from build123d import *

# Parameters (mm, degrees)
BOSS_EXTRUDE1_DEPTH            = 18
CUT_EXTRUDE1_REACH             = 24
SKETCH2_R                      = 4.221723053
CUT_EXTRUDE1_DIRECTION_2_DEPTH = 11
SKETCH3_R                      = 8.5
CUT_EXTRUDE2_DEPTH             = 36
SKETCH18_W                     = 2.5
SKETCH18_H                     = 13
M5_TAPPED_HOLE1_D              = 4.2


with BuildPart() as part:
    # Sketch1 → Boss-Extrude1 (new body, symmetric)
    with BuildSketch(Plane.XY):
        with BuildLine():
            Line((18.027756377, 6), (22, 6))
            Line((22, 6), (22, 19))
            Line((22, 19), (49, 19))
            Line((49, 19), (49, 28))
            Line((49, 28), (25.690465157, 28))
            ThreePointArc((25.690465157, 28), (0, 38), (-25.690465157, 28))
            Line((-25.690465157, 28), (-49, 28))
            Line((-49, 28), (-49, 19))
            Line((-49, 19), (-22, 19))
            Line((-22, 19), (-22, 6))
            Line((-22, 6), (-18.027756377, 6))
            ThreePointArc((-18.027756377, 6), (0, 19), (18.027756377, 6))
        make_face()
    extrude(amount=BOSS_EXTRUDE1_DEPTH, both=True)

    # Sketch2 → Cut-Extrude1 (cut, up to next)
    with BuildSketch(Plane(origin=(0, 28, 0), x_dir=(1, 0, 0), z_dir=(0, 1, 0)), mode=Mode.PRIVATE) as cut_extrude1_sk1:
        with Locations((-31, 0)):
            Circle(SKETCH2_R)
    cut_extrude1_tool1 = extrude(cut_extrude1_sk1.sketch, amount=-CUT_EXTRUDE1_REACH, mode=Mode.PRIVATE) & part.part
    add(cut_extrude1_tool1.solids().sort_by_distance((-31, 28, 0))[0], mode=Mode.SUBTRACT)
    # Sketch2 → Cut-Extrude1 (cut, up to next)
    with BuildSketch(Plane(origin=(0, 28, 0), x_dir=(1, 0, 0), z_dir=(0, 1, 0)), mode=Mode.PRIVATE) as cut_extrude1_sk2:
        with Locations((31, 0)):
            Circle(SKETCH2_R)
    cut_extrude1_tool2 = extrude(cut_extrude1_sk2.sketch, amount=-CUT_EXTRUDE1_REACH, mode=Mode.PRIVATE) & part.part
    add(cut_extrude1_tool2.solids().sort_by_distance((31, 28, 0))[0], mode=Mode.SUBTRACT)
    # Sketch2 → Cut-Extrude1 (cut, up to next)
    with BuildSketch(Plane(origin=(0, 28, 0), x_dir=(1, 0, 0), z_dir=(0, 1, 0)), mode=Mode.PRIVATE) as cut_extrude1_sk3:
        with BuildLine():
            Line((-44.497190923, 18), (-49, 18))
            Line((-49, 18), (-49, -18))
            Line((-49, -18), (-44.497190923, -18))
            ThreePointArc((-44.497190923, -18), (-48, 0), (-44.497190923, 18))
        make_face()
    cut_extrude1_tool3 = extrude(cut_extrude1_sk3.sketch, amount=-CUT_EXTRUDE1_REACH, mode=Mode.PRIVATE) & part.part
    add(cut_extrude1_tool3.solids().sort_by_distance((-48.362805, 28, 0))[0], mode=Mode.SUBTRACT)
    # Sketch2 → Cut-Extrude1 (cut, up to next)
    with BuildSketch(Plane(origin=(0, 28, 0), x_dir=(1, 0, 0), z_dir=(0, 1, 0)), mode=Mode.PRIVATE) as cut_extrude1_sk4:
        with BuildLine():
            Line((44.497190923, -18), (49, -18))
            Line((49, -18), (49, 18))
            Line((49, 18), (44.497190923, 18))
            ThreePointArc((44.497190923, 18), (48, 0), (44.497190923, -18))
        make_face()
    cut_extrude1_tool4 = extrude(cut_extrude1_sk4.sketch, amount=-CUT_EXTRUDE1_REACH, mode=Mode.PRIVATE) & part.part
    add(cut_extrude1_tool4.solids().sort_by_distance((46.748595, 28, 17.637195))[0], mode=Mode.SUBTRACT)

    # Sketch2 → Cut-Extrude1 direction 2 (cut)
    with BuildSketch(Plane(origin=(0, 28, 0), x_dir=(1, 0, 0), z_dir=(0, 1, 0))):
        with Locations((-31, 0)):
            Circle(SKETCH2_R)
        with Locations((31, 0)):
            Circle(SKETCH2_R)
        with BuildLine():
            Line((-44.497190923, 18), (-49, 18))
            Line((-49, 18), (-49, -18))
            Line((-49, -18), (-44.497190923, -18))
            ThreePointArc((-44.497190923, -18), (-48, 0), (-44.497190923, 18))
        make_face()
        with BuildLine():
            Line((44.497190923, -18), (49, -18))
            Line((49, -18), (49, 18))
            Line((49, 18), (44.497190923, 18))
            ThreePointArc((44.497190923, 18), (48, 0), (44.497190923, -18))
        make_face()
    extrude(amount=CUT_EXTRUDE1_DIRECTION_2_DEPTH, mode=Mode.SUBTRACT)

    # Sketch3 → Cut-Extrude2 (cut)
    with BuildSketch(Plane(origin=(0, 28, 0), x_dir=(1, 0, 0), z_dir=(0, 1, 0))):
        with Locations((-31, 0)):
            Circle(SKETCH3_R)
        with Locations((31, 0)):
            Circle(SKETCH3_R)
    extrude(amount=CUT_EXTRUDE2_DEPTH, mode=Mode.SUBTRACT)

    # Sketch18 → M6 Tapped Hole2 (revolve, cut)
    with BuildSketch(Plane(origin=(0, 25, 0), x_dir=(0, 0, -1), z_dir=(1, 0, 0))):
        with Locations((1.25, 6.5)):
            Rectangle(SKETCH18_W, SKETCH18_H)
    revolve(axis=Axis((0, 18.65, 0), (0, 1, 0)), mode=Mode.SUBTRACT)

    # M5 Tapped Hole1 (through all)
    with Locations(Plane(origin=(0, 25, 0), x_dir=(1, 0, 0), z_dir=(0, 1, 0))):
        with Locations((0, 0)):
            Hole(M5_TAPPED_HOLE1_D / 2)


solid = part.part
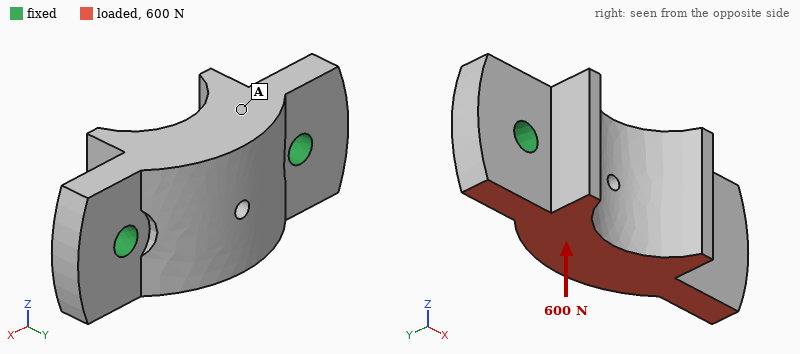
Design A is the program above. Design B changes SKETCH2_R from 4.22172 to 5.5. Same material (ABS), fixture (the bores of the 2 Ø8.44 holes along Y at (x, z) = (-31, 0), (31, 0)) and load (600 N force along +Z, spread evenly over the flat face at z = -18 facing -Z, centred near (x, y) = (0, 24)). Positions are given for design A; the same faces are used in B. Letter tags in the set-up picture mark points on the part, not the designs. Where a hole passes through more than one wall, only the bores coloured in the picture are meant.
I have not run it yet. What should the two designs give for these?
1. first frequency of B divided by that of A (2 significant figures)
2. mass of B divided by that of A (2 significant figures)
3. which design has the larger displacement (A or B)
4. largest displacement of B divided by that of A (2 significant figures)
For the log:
1.2
0.99
A
0.85
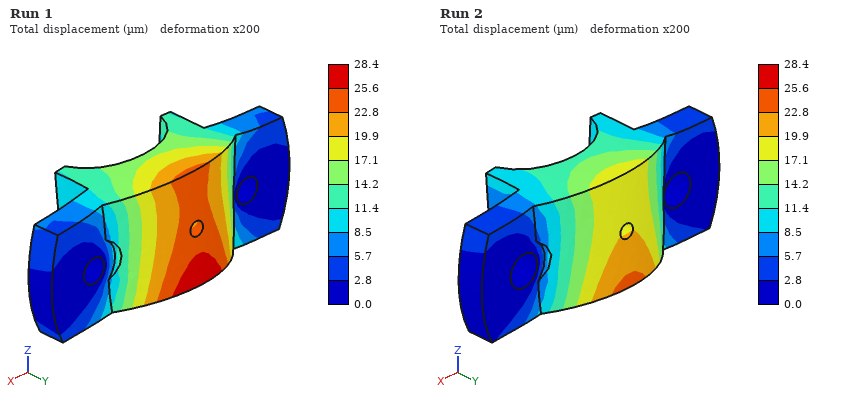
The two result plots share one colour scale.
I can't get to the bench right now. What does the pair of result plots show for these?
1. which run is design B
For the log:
Run 2
